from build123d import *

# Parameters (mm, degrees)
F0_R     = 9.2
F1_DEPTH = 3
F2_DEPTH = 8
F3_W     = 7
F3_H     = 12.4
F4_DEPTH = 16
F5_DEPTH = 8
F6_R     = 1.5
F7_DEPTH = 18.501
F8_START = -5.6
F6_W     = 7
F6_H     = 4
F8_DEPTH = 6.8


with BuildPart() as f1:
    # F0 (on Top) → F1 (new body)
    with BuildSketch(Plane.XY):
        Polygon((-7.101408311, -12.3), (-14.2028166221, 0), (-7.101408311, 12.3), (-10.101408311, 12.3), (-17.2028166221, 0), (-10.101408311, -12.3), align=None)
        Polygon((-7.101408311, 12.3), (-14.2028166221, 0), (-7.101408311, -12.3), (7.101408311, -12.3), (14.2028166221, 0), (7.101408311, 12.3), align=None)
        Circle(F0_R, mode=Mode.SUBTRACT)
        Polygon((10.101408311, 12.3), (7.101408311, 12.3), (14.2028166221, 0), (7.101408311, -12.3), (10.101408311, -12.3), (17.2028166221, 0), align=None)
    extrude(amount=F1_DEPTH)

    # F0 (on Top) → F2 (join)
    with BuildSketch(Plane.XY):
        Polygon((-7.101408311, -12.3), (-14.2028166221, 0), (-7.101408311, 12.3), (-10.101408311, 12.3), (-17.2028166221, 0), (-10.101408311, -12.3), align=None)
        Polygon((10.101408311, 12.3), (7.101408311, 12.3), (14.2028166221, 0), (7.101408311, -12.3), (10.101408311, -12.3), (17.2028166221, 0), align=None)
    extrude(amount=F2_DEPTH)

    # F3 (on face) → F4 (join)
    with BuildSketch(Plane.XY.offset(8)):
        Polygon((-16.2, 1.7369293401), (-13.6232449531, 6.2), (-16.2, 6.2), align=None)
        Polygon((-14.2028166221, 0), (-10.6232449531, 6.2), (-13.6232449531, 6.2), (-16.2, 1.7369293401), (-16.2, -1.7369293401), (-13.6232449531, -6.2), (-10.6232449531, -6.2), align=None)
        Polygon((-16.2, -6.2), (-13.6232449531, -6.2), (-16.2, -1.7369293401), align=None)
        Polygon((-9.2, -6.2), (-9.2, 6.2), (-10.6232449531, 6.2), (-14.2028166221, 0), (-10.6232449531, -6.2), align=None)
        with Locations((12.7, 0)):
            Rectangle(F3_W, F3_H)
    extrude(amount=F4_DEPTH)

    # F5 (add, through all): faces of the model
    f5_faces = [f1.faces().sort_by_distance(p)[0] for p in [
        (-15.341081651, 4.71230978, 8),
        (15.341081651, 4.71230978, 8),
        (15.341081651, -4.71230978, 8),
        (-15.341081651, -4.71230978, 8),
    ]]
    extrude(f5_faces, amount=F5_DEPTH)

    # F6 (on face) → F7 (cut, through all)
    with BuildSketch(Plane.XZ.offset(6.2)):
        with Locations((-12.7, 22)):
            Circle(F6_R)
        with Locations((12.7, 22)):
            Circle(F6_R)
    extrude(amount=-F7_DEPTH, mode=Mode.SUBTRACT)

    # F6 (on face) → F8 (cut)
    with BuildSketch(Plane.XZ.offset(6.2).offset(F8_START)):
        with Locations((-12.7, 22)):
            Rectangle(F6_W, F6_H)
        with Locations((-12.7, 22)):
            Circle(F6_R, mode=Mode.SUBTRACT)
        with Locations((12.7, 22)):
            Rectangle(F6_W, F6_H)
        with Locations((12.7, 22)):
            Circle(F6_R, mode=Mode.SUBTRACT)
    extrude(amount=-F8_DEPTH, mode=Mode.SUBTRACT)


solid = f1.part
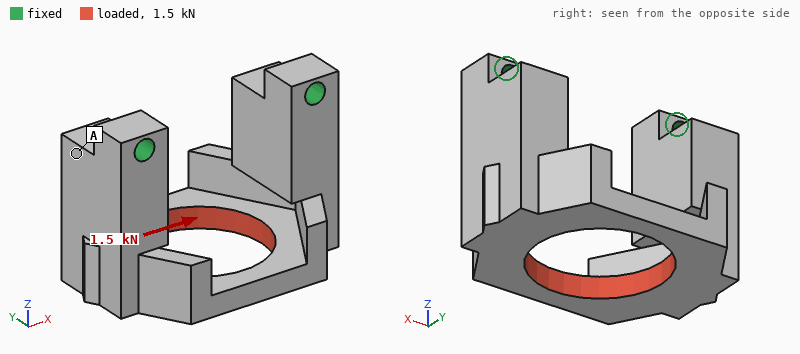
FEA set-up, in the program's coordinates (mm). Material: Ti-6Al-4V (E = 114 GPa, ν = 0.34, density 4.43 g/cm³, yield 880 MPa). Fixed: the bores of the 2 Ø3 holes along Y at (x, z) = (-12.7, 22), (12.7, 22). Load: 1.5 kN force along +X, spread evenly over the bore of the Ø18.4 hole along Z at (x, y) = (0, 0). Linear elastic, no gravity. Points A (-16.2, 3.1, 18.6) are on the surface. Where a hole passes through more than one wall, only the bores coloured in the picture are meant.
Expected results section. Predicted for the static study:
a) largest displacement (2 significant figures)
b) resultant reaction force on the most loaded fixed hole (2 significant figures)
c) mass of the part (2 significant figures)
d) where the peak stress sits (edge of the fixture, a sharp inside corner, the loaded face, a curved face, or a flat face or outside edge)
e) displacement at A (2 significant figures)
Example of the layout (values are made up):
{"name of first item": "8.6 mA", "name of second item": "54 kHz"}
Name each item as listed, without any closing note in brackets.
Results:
{"largest displacement": "94 µm", "resultant reaction force on the most loaded fixed hole": "820 N", "mass of the part": "20 g", "where the peak stress sits": "edge of the fixture", "displacement at A": "17 µm"}
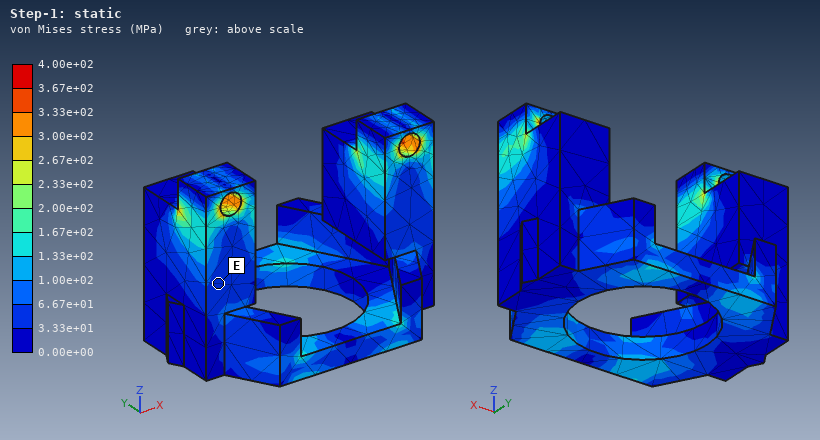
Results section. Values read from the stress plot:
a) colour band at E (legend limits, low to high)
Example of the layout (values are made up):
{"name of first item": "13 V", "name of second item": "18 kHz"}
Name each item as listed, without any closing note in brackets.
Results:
{"colour band at E": "3.33e+01 to 6.67e+01 MPa"}
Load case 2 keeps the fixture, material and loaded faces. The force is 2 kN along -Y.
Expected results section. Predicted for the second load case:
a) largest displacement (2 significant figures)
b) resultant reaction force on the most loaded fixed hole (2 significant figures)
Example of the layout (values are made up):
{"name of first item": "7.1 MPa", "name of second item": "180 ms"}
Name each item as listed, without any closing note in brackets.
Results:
{"largest displacement": "0.20 mm", "resultant reaction force on the most loaded fixed hole": "1.0 kN"}
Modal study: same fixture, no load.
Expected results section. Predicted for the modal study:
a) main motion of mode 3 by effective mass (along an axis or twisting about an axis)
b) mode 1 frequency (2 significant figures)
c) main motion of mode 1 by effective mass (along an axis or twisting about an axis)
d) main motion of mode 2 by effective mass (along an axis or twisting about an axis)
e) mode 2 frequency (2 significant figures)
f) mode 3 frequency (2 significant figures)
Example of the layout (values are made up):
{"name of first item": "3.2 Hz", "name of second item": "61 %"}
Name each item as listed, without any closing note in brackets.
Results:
{"main motion of mode 3 by effective mass": "twisting about Z", "mode 1 frequency": "5700 Hz", "main motion of mode 1 by effective mass": "along Y", "main motion of mode 2 by effective mass": "along X", "mode 2 frequency": "6800 Hz", "mode 3 frequency": "8500 Hz"}
